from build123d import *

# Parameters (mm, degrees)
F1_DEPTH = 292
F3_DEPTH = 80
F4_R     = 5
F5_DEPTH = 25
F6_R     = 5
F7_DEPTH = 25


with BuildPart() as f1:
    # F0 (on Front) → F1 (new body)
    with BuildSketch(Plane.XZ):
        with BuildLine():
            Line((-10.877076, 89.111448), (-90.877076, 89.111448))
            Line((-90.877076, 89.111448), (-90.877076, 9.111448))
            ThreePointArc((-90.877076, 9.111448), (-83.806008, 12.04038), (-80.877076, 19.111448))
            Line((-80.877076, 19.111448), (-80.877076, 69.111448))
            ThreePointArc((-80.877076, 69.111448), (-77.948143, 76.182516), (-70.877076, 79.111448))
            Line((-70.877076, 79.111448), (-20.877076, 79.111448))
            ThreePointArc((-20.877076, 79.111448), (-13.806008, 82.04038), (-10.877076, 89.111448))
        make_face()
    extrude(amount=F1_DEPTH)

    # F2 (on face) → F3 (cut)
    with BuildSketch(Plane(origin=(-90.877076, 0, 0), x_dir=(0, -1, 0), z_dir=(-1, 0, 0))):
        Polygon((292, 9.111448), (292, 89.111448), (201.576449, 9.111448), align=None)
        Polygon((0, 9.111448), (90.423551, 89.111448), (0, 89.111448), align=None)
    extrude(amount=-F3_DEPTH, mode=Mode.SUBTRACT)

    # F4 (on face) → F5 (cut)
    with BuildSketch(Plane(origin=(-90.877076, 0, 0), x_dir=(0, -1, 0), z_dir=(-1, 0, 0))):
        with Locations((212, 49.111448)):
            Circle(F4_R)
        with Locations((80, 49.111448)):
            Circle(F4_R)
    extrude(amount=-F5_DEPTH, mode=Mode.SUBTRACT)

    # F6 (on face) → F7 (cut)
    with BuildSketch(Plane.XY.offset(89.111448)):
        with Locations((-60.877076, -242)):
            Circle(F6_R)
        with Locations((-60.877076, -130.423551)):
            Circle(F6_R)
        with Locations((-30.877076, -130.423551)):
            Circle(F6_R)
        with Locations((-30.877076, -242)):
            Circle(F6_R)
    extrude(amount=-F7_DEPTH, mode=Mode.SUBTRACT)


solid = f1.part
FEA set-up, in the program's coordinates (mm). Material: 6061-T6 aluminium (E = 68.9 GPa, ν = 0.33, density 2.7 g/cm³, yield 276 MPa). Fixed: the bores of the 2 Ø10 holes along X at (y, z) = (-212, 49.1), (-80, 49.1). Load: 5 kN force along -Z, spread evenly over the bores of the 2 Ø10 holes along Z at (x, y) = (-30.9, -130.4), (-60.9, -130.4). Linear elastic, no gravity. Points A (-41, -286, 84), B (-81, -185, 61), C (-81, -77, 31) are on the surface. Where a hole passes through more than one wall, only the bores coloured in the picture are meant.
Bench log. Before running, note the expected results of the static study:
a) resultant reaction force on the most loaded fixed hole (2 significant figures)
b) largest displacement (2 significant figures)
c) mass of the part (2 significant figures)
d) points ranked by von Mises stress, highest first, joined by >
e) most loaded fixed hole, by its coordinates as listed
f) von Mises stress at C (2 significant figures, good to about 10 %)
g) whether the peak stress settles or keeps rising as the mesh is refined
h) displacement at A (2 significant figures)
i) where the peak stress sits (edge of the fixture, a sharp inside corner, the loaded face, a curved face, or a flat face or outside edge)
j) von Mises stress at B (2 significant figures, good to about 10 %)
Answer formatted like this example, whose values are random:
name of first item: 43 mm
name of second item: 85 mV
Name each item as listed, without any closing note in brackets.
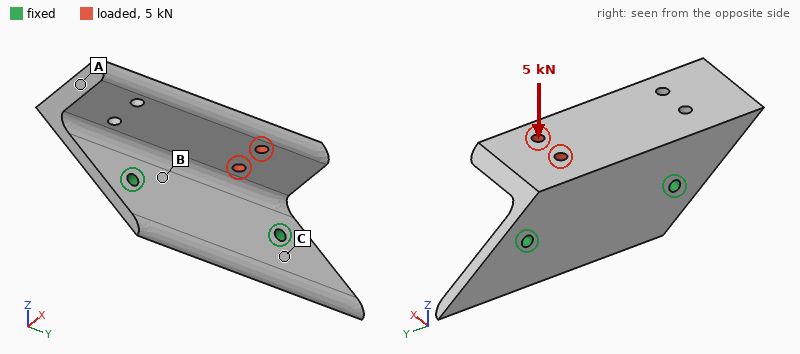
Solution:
resultant reaction force on the most loaded fixed hole: 3.1 kN
largest displacement: 0.92 mm
mass of the part: 790 g
points ranked by von Mises stress, highest first, joined by >: B > C > A
most loaded fixed hole, by its coordinates as listed: (-80, 49.1)
von Mises stress at C: 28 MPa
whether the peak stress settles or keeps rising as the mesh is refined: keeps rising
displacement at A: 0.23 mm
where the peak stress sits: edge of the fixture
von Mises stress at B: 50 MPa
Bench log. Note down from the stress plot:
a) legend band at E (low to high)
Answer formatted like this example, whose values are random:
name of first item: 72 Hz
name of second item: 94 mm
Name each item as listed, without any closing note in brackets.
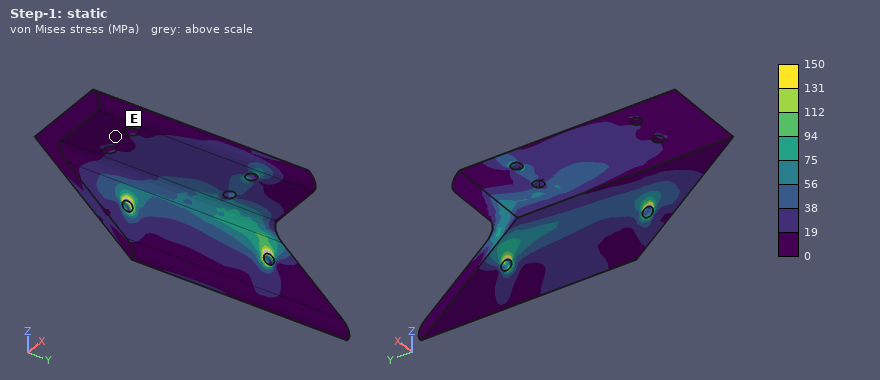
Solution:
legend band at E: 0 to 19 MPa
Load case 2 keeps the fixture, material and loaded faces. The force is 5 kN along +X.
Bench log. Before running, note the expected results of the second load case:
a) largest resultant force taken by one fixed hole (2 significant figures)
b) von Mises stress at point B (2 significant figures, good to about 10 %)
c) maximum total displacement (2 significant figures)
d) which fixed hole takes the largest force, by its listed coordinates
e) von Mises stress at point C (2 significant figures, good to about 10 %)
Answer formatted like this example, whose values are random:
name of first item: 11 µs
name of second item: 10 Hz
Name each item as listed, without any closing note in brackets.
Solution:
largest resultant force taken by one fixed hole: 3.2 kN
von Mises stress at point B: 22 MPa
maximum total displacement: 0.39 mm
which fixed hole takes the largest force, by its listed coordinates: (-80, 49.1)
von Mises stress at point C: 14 MPa
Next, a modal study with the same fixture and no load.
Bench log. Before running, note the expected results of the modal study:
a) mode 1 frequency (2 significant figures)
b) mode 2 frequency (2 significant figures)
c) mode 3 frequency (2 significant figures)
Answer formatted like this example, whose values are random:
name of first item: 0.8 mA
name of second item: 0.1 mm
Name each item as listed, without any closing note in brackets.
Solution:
mode 1 frequency: 770 Hz
mode 2 frequency: 1300 Hz
mode 3 frequency: 2000 Hz
